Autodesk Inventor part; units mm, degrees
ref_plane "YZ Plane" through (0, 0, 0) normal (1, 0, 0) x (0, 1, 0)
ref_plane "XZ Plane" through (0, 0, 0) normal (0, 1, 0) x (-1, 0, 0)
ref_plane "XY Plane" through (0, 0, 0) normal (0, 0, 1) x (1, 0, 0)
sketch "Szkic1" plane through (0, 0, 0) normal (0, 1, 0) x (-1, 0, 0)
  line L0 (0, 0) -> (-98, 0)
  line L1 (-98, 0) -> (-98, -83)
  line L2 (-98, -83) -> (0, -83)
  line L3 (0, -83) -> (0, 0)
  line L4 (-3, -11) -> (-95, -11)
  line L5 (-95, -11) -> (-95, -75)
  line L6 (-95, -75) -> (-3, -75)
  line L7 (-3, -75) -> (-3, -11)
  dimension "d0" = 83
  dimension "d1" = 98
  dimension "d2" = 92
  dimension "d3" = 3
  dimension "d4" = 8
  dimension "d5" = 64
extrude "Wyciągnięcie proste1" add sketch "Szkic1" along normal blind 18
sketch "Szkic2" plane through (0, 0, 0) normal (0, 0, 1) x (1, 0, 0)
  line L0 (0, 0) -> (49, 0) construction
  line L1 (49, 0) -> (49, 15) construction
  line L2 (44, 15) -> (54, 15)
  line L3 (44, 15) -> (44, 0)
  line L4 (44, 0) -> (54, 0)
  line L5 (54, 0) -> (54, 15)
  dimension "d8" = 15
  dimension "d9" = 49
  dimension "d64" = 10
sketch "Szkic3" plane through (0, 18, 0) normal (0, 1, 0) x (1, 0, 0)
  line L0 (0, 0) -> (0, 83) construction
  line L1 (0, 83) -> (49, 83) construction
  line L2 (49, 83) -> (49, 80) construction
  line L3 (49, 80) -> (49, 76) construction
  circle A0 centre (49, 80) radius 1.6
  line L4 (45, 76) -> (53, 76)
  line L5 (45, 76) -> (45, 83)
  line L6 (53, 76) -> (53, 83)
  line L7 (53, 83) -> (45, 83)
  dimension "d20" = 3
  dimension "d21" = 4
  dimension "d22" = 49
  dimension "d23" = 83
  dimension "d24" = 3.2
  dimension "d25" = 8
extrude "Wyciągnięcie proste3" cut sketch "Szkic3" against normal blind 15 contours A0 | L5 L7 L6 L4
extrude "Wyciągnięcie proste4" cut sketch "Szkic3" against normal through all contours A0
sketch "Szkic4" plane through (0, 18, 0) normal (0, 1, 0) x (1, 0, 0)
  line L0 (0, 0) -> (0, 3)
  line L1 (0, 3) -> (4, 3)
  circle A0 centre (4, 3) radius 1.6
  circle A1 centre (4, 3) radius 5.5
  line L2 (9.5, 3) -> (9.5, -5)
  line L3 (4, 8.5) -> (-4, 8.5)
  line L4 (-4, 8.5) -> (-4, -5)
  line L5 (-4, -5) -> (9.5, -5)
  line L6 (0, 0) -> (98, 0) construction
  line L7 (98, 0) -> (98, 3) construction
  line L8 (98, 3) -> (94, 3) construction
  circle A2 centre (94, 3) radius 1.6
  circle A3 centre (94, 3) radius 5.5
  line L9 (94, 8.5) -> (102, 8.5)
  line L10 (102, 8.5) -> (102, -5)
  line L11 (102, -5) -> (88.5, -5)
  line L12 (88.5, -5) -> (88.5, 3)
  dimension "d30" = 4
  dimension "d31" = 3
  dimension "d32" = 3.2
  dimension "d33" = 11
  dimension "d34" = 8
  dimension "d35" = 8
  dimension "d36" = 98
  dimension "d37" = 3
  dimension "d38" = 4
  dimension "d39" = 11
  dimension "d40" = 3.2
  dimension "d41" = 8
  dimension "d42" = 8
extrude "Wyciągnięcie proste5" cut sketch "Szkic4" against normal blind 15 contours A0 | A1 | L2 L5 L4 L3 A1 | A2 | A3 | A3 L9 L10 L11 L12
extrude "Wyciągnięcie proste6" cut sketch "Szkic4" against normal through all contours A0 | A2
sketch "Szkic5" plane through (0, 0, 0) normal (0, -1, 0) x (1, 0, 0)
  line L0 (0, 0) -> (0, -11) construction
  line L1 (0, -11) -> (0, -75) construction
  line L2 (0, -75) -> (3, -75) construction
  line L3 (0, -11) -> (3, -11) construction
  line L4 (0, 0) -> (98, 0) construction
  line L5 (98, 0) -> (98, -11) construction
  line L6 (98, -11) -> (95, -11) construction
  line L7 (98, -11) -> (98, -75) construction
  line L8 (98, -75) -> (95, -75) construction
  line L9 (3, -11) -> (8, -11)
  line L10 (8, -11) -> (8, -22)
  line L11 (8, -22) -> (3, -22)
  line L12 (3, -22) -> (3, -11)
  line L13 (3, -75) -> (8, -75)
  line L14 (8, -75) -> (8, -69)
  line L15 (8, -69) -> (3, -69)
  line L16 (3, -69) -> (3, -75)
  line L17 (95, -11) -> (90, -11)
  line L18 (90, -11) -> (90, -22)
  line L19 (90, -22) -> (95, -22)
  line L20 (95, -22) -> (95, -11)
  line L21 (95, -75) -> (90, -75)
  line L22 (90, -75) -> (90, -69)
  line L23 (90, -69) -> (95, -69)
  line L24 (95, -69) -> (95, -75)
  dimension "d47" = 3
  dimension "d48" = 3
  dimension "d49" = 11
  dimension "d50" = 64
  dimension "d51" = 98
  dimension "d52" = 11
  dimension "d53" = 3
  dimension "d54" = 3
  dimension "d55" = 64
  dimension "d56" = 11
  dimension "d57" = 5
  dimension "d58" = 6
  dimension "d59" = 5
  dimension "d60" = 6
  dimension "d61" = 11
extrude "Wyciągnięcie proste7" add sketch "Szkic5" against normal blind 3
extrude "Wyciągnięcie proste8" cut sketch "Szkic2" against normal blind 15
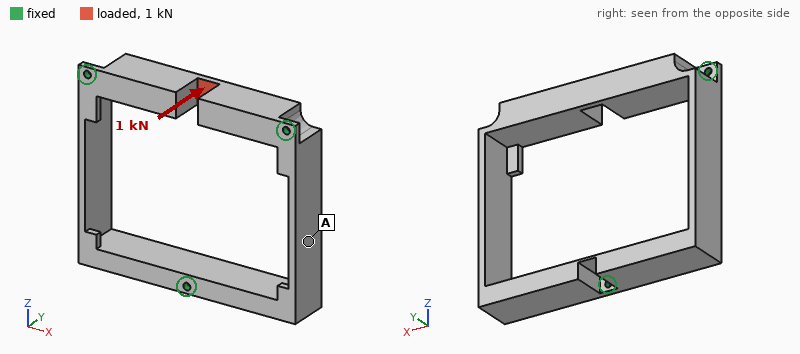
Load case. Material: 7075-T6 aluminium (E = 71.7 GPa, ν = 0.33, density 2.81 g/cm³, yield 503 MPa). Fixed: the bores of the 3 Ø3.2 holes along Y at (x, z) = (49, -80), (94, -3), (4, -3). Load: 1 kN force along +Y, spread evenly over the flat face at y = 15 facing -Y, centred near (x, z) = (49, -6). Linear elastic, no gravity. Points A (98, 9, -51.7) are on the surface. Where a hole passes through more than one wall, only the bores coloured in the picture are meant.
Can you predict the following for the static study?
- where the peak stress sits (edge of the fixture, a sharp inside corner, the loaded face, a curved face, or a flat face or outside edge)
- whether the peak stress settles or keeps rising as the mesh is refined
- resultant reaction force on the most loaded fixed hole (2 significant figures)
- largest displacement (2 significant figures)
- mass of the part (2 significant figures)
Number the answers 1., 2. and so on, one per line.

1. edge of the fixture
2. keeps rising
3. 1.4 kN
4. 56 µm
5. 100 g
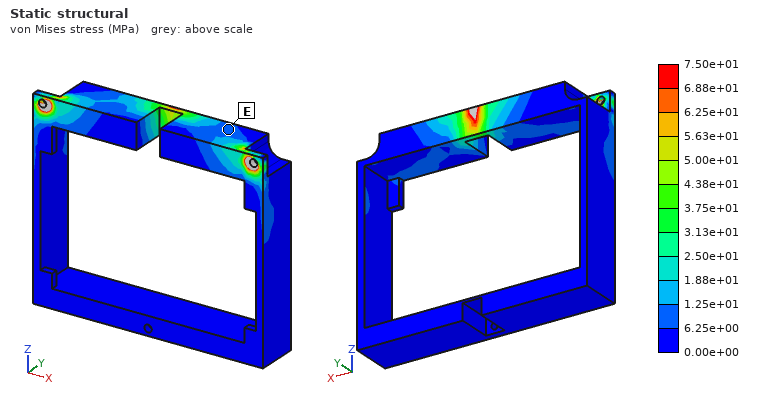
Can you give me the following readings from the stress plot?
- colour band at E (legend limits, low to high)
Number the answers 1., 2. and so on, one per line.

1. 6.25e+00 to 1.25e+01 MPa
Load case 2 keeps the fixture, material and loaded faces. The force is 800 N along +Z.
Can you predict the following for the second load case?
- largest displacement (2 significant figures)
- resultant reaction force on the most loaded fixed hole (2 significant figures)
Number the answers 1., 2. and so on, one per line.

1. 0.20 mm
2. 400 N
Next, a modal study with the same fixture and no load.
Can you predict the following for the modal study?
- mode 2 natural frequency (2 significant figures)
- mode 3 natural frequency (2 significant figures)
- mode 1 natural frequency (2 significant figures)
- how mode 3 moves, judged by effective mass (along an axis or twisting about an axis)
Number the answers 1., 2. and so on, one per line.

1. 2500 Hz
2. 3000 Hz
3. 1200 Hz
4. along Y
